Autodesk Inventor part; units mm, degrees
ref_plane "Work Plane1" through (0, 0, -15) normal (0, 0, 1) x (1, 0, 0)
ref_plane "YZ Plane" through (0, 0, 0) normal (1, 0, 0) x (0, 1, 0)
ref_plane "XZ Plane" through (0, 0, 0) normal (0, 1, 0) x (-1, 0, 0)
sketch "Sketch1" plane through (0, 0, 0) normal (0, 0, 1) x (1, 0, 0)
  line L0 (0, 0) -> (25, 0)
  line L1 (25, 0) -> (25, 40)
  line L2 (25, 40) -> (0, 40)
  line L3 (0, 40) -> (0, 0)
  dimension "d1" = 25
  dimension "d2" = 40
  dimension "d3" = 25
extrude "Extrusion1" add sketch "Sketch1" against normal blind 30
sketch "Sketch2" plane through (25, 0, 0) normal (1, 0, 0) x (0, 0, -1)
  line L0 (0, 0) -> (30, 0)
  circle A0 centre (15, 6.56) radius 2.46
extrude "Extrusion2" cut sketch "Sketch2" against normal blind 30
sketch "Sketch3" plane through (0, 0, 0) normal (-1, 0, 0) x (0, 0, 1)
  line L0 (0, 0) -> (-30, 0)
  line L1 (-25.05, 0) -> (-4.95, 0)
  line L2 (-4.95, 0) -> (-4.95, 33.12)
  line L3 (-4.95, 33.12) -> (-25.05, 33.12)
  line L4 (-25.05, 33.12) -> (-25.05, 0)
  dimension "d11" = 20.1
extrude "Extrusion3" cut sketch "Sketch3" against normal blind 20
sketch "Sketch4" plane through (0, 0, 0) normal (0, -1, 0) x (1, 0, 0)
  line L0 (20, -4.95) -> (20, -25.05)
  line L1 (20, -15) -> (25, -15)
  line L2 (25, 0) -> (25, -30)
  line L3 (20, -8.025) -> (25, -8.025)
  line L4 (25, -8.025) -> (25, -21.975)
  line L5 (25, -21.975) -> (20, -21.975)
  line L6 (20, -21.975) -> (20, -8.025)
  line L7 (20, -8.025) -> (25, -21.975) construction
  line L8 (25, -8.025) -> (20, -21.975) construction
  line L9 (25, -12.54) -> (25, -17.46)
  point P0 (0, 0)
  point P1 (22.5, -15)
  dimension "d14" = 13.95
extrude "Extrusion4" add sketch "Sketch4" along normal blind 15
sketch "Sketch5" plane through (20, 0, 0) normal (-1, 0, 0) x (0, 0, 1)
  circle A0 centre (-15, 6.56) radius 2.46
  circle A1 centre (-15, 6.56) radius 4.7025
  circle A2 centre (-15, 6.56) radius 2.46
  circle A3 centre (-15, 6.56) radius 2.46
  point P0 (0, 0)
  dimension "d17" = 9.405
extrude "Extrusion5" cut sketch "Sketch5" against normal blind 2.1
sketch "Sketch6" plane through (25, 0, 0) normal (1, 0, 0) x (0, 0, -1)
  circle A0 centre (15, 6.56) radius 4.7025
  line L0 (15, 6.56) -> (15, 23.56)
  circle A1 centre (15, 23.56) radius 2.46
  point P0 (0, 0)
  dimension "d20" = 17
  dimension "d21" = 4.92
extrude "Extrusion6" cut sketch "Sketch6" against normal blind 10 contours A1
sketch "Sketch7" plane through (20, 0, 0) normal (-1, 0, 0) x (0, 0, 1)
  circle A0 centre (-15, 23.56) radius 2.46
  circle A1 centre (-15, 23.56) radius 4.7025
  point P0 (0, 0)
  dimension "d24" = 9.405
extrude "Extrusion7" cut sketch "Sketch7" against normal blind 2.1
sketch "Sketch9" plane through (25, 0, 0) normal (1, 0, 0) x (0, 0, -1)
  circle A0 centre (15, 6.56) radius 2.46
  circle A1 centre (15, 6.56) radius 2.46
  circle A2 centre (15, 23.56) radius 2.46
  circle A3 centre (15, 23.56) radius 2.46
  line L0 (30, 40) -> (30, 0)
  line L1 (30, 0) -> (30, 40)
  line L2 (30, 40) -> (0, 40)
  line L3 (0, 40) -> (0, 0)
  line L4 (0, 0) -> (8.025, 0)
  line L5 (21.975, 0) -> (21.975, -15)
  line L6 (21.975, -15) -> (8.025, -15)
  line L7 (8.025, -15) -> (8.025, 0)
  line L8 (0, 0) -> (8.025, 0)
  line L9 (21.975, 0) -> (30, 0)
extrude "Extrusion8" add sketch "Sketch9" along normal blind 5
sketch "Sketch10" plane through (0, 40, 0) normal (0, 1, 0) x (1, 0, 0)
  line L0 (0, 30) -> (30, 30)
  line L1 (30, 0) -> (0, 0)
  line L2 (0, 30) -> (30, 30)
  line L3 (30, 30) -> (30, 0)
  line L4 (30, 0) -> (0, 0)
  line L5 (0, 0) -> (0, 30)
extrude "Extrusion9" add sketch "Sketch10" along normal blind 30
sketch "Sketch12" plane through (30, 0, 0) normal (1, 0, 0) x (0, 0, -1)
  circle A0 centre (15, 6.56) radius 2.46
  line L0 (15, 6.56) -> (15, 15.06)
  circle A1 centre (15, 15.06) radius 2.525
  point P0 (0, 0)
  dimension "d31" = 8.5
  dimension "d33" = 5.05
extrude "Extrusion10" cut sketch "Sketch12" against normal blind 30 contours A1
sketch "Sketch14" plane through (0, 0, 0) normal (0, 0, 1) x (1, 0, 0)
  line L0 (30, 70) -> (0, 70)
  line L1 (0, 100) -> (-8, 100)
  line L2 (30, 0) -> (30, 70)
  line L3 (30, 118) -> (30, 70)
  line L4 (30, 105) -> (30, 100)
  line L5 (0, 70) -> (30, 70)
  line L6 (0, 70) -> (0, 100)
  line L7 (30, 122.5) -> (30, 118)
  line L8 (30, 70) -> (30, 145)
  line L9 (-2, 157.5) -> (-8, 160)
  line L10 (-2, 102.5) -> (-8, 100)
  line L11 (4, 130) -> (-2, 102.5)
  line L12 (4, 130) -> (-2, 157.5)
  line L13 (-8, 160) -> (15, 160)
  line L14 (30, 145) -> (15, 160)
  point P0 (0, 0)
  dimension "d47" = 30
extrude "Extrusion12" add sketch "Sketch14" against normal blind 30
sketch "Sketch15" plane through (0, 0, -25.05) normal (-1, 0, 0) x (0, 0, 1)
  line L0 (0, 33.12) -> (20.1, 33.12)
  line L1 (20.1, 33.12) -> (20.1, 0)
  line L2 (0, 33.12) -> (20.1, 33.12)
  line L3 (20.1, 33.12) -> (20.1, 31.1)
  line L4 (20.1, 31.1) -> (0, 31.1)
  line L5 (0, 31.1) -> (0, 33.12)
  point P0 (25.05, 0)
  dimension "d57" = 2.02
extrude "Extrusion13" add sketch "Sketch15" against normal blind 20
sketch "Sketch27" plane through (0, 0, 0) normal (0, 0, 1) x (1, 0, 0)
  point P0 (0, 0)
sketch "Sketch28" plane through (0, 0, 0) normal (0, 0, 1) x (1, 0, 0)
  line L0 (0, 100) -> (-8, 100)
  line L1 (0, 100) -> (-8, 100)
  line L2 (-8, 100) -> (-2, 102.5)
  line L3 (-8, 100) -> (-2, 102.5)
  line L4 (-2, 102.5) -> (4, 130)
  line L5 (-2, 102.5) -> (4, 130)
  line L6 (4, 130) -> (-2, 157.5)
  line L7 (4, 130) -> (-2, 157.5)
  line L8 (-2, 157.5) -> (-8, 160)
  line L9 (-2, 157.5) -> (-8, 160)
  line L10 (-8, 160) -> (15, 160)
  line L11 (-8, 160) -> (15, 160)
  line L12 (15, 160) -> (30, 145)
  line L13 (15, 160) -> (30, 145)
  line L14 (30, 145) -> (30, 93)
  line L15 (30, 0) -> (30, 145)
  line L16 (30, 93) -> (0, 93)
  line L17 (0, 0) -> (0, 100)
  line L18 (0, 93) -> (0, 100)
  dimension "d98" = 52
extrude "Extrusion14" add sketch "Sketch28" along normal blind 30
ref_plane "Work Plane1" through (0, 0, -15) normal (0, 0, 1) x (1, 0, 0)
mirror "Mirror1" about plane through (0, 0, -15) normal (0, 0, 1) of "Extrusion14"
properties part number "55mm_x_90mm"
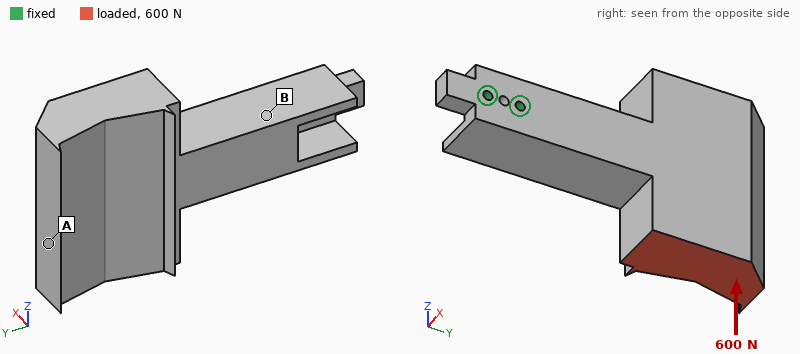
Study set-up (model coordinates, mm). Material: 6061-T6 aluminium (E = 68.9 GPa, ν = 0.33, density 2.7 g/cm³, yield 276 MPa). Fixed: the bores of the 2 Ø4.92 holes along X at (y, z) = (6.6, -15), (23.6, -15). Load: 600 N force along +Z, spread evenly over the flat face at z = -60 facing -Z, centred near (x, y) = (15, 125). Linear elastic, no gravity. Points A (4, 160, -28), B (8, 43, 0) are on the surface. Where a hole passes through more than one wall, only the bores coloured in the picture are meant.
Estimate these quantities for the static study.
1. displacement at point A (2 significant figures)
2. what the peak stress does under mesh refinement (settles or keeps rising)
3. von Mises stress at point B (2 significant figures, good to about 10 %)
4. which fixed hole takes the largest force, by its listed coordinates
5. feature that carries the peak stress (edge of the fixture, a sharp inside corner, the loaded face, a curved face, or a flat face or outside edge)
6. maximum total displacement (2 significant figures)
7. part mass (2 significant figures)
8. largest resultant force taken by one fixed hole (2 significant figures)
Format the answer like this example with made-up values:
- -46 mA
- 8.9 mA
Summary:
- 0.18 mm
- keeps rising
- 9.6 MPa
- (23.6, -15)
- edge of the fixture
- 0.19 mm
- 650 g
- 3.2 kN
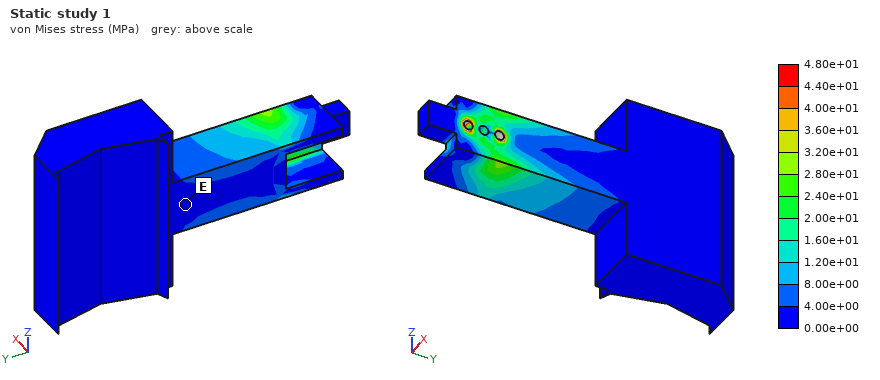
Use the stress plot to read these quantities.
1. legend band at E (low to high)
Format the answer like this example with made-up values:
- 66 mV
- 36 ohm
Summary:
- 0.00e+00 to 4.00e+00 MPa
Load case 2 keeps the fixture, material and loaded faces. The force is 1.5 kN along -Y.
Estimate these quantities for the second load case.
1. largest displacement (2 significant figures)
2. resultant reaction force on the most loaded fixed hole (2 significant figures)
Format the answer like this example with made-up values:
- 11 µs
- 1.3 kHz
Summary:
- 0.27 mm
- 3.1 kN
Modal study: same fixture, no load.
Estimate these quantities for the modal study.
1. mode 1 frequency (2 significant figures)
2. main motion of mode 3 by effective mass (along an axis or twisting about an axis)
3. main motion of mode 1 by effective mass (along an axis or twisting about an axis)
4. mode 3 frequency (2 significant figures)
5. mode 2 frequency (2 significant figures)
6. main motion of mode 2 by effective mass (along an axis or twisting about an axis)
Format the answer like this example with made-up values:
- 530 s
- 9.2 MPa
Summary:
- 420 Hz
- twisting about Y
- along X
- 1000 Hz
- 470 Hz
- along Z
